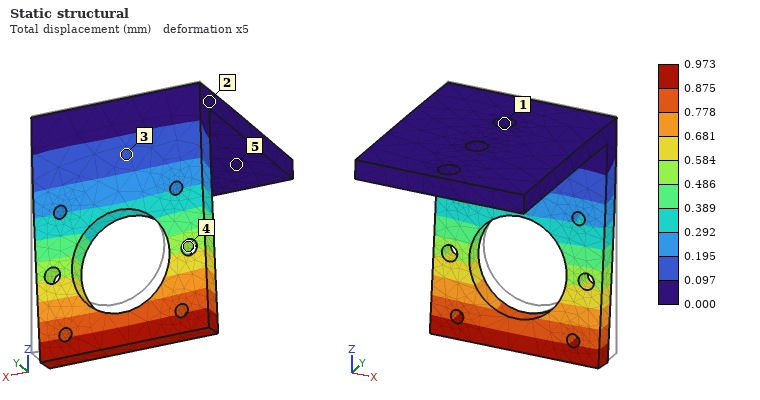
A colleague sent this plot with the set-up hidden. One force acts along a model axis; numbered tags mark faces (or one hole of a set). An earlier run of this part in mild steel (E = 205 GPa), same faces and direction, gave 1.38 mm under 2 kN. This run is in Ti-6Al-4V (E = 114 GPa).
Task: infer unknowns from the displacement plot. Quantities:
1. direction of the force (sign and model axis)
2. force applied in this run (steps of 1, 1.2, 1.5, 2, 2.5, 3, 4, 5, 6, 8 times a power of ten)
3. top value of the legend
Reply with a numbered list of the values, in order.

1. -Y
2. 800 N
3. 0.973 mm
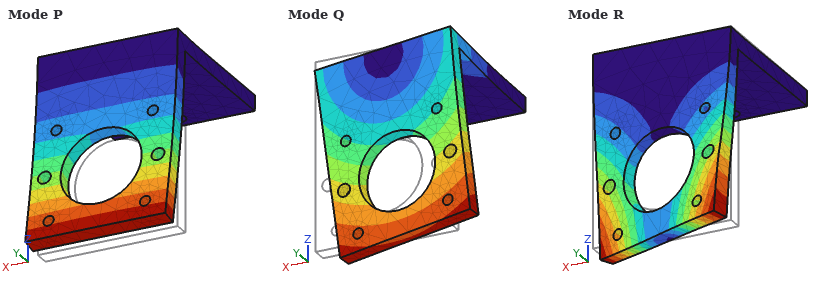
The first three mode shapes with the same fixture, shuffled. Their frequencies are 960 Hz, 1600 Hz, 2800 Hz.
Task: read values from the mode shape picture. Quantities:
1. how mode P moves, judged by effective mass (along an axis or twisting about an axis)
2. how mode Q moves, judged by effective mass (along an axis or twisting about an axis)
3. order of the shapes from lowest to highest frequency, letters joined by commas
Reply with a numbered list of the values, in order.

1. along Y
2. along X
3. P, Q, R
